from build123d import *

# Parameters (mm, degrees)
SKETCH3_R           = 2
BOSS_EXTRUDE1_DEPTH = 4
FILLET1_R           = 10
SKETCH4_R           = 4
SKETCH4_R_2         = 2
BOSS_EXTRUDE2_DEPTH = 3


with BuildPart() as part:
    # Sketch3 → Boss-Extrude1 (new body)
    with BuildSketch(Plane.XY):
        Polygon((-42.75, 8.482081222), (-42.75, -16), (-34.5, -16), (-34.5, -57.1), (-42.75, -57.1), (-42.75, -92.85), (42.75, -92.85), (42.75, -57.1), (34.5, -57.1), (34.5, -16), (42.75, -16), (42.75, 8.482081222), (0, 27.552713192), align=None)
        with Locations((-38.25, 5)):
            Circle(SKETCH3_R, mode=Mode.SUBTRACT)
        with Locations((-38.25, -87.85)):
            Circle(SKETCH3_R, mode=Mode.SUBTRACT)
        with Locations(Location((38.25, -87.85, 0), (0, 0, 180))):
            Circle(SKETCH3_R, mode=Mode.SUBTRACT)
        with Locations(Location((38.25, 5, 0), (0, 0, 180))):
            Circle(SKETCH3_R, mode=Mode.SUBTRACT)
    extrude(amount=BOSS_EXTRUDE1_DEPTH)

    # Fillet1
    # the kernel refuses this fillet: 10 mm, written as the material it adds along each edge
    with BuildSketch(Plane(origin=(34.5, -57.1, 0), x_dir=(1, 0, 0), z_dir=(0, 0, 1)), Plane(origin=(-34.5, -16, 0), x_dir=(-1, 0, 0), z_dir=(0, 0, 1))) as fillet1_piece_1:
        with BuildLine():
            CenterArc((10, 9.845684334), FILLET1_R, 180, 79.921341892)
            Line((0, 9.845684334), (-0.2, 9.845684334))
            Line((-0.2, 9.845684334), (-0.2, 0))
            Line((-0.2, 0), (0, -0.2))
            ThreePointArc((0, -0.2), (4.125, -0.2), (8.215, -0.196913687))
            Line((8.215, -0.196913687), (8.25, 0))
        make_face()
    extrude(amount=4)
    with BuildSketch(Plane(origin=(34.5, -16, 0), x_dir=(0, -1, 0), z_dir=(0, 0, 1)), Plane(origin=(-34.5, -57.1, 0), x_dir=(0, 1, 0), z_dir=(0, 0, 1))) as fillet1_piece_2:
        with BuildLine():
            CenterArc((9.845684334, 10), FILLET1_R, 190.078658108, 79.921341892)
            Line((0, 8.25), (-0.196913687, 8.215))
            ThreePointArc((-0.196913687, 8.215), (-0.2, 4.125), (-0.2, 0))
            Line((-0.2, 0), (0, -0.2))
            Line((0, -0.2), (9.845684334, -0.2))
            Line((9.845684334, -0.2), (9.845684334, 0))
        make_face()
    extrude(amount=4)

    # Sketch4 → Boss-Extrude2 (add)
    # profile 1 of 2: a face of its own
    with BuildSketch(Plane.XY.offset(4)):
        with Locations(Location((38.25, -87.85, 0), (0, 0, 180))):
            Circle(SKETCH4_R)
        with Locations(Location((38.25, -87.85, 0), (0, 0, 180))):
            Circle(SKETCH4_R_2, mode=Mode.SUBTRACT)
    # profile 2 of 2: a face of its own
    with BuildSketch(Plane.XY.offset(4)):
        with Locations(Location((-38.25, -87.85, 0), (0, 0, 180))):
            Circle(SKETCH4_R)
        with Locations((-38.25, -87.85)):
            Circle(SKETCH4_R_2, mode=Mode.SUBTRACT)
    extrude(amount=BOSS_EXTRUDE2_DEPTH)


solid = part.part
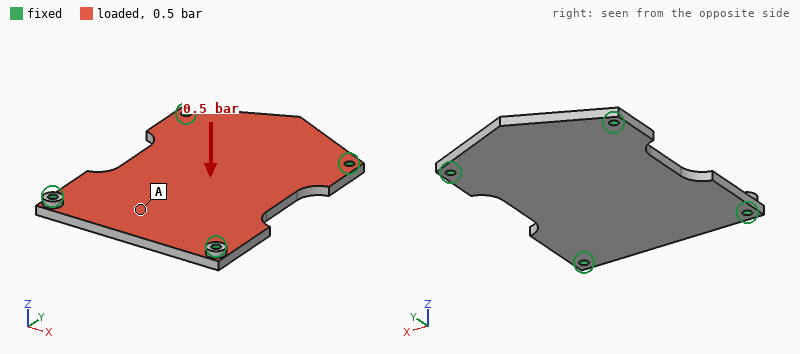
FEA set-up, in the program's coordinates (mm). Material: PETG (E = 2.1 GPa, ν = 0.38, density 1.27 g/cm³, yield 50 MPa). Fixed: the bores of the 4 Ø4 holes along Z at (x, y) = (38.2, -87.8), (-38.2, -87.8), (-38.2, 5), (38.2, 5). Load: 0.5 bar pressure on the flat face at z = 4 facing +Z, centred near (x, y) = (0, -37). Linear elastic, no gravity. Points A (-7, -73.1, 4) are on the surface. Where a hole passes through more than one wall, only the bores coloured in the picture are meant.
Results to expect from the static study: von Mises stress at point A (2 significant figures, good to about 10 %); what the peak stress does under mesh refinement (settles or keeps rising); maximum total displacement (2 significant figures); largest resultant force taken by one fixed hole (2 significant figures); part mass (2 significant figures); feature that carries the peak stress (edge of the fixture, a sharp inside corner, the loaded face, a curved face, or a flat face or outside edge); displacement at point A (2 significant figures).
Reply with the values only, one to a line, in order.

5.5 MPa
keeps rising
1.7 mm
120 N
45 g
edge of the fixture
0.99 mm
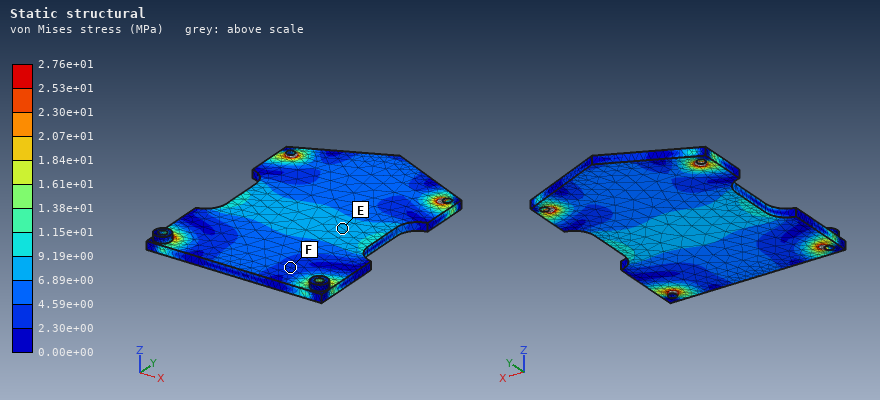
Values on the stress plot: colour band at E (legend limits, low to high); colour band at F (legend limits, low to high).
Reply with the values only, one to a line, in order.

6.89e+00 to 9.19e+00 MPa
2.30e+00 to 4.59e+00 MPa
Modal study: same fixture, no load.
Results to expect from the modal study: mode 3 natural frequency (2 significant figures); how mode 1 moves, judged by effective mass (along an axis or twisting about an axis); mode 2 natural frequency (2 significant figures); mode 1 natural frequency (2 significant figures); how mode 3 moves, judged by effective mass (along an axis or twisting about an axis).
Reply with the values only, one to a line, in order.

830 Hz
along Z
760 Hz
450 Hz
twisting about Y
